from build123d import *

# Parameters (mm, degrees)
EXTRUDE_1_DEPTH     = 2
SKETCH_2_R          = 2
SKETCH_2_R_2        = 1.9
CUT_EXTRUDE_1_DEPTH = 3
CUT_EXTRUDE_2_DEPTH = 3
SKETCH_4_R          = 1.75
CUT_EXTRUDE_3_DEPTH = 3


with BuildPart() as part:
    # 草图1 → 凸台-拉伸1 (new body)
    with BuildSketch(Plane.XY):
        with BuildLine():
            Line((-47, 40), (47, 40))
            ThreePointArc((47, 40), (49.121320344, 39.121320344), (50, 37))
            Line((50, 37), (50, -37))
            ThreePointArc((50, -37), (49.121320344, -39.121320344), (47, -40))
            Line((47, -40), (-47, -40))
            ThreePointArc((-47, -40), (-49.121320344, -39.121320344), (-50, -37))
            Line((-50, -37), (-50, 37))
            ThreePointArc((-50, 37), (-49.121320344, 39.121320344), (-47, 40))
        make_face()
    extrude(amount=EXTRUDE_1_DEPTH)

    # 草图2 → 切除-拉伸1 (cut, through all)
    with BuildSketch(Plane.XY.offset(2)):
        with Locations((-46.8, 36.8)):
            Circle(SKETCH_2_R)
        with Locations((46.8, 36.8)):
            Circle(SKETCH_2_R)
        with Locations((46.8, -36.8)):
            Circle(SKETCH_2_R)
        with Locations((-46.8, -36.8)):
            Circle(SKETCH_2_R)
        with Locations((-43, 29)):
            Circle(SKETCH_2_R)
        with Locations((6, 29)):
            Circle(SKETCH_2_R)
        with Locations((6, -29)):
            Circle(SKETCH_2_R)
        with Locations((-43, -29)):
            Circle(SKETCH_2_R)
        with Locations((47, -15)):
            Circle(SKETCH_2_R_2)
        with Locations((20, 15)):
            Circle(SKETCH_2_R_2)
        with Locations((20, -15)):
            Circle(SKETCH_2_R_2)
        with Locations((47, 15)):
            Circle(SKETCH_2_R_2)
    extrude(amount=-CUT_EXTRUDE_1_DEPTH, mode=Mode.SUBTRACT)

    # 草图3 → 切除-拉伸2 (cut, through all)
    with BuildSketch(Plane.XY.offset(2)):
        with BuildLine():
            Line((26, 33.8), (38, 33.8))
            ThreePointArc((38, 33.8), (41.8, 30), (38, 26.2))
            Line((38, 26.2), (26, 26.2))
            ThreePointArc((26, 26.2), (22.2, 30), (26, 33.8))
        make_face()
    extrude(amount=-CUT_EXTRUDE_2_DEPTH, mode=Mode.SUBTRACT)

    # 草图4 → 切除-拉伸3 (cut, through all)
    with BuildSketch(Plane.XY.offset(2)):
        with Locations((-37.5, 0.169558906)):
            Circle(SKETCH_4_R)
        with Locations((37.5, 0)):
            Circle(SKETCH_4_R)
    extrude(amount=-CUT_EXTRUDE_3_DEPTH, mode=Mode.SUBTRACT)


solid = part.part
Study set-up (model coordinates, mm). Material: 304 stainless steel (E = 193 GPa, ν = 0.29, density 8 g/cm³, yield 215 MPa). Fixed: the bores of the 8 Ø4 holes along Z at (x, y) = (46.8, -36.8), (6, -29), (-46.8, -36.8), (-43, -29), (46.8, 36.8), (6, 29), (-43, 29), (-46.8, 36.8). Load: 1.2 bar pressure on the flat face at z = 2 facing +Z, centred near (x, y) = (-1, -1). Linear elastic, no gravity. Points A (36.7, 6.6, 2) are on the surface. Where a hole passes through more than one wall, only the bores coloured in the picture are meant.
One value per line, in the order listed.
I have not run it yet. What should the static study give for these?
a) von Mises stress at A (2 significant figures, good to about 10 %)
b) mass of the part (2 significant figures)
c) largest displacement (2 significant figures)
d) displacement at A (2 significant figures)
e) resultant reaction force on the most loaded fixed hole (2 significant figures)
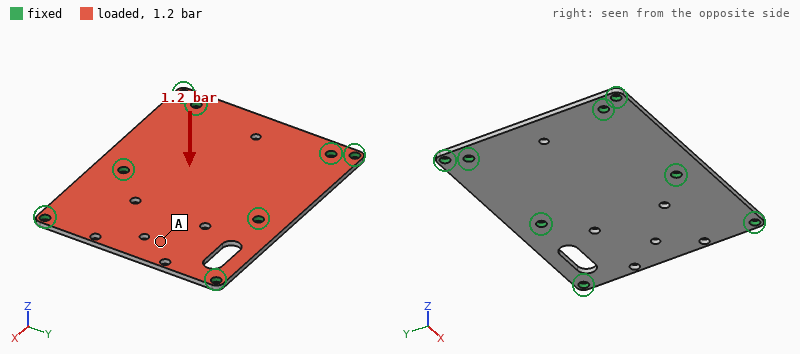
27 MPa
120 g
77 µm
63 µm
230 N
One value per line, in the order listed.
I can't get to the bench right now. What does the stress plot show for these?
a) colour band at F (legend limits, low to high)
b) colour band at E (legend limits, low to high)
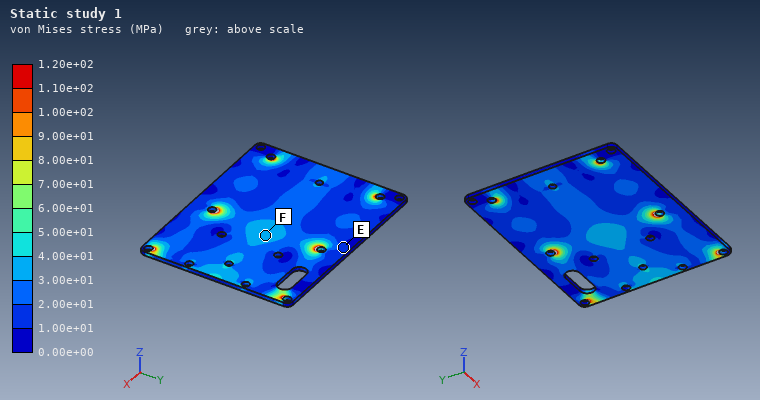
3.00e+01 to 4.00e+01 MPa
1.00e+01 to 2.00e+01 MPa
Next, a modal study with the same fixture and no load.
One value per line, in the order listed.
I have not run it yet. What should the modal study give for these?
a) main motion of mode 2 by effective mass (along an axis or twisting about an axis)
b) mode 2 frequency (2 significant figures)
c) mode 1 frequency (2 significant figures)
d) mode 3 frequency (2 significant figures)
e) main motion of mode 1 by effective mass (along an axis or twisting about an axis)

along Z
2500 Hz
2000 Hz
3800 Hz
along Z
